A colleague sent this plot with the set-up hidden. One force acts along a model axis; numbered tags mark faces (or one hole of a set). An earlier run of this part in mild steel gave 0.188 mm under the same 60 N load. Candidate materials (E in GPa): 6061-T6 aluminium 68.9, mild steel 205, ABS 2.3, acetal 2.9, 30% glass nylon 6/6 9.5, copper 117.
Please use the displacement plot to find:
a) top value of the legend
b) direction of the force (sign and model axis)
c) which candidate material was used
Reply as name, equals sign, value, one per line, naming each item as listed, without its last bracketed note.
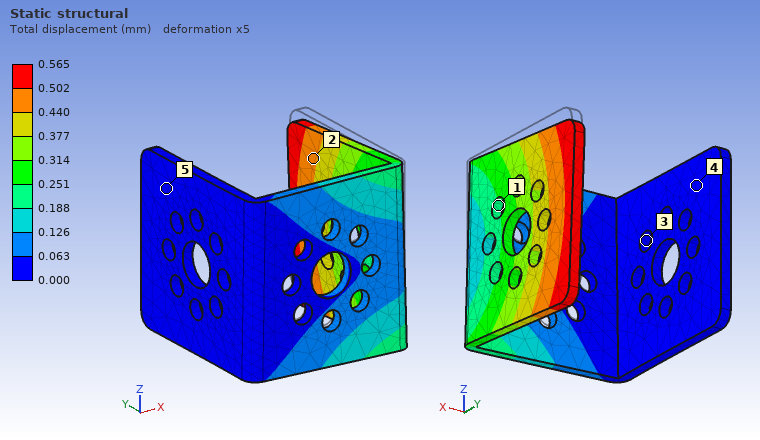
top value of the legend = 0.565 mm
direction of the force = -Z
which candidate material was used = 6061-T6 aluminium
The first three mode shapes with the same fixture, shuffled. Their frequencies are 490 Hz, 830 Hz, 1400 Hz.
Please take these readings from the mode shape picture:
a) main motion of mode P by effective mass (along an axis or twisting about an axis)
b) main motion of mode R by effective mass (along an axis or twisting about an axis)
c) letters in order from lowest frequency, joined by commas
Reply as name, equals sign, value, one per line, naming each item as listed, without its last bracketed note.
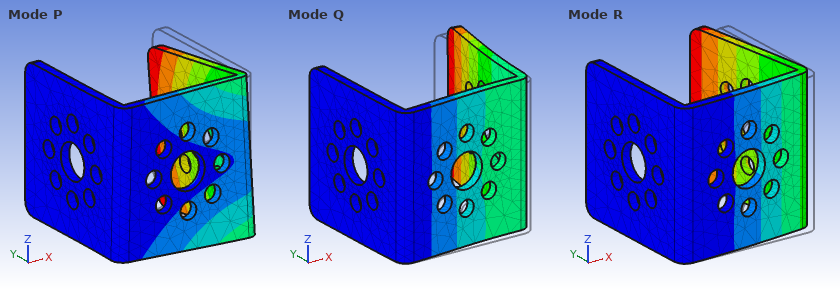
main motion of mode P by effective mass = along Z
main motion of mode R by effective mass = along Y
letters in order from lowest frequency, joined by commas = R, P, Q
